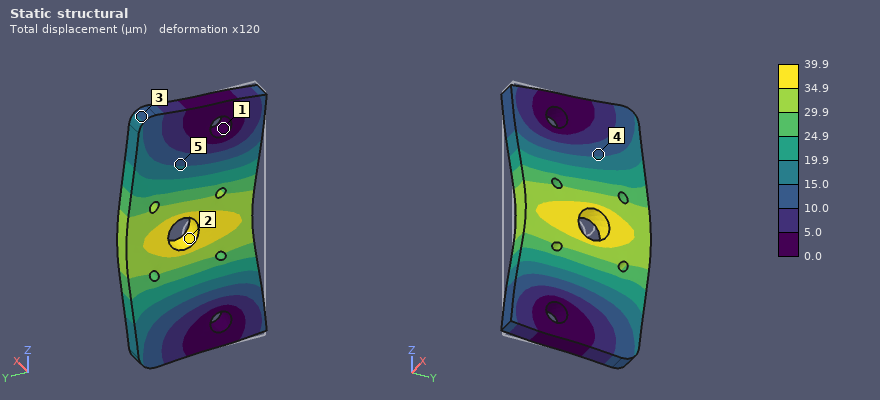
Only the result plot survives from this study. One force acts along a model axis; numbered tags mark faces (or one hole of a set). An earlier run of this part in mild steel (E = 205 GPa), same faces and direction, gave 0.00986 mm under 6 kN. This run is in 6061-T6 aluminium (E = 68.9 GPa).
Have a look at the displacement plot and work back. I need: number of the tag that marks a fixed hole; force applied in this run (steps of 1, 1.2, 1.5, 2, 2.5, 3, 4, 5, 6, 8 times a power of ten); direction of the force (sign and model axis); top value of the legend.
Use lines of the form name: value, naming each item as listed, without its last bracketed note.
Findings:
number of the tag that marks a fixed hole: 1
force applied in this run: 8 kN
direction of the force: +Y
top value of the legend: 39.9 µm
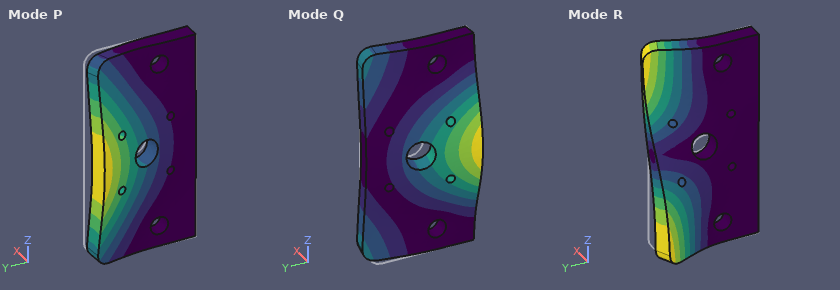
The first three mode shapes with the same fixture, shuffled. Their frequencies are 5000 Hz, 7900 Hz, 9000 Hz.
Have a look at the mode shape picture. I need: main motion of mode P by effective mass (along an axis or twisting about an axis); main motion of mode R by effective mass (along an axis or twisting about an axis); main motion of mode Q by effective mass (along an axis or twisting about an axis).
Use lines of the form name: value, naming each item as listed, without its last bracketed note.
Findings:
main motion of mode P by effective mass: along X
main motion of mode R by effective mass: twisting about Y
main motion of mode Q by effective mass: along X
